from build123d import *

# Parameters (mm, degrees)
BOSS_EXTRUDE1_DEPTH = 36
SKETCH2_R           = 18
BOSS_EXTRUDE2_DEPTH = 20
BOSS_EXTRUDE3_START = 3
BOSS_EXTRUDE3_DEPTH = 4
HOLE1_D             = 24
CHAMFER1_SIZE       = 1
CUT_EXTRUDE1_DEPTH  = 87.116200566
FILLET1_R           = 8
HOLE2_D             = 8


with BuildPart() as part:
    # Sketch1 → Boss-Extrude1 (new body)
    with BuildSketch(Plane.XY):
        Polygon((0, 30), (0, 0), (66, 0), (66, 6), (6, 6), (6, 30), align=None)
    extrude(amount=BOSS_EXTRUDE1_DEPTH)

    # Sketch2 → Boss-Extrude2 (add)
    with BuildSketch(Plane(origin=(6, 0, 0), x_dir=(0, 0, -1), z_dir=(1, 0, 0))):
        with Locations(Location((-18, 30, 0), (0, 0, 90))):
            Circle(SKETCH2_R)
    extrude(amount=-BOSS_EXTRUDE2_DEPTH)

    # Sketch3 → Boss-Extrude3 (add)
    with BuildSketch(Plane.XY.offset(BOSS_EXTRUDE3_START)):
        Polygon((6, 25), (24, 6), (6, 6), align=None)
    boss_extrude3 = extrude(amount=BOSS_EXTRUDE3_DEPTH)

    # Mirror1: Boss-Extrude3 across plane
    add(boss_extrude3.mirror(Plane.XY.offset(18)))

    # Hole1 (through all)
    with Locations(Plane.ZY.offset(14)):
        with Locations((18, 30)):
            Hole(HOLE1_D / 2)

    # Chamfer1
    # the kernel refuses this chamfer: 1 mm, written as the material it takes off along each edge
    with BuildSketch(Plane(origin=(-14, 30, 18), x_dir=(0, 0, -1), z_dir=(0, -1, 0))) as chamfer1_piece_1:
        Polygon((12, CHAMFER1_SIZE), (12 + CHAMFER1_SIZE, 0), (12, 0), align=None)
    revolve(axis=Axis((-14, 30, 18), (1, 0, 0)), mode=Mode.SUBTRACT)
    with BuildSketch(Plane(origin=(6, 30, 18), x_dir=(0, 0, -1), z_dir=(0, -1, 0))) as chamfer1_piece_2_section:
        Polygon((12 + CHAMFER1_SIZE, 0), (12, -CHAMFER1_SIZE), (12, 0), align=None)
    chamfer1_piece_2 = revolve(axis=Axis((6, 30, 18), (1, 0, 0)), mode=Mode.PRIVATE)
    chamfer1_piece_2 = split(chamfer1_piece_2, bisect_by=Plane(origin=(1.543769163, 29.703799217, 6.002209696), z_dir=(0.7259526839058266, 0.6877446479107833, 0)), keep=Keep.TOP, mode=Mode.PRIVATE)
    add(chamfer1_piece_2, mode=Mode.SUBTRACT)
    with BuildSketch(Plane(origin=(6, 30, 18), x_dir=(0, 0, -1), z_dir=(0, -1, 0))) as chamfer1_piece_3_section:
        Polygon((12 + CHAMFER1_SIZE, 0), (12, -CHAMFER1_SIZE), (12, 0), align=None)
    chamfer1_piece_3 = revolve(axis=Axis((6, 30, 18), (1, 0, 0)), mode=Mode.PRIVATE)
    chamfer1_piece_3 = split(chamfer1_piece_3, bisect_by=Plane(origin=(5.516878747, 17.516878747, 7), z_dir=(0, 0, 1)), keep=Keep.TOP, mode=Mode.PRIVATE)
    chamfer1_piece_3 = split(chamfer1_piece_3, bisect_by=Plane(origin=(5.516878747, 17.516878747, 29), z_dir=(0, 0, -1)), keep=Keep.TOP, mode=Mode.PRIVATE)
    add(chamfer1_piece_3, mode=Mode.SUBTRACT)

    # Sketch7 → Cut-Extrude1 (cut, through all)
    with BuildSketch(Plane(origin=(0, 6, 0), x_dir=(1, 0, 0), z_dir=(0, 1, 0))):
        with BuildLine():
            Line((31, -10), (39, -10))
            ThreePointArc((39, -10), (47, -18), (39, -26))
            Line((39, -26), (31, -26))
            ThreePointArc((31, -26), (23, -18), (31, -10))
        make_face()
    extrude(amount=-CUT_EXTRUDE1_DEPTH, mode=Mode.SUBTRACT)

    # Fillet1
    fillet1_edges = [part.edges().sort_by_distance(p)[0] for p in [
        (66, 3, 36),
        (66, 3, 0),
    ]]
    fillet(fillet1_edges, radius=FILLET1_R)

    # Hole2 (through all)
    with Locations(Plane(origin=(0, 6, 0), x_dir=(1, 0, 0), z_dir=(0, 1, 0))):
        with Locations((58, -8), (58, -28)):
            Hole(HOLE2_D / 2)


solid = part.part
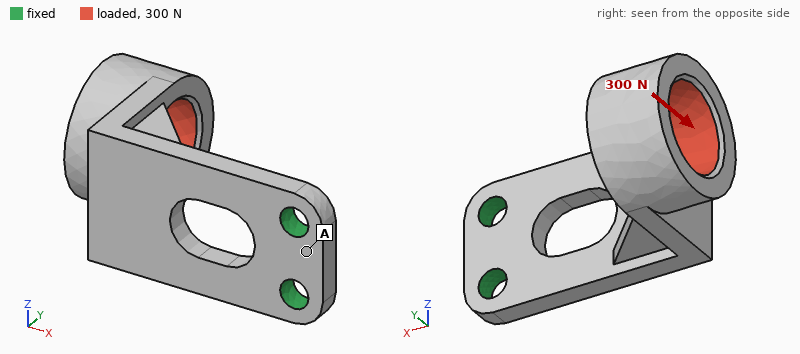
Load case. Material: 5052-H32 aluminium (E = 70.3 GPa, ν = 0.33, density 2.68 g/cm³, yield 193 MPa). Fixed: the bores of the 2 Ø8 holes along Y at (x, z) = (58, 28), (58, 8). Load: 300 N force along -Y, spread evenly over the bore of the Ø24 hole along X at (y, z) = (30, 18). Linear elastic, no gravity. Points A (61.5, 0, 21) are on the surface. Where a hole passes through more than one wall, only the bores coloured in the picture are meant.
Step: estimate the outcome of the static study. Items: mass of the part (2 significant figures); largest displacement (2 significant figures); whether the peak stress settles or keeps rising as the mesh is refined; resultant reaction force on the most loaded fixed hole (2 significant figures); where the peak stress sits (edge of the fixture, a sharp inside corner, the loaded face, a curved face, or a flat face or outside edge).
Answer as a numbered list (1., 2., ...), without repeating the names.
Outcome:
1. 70 g
2. 1.0 mm
3. keeps rising
4. 150 N
5. edge of the fixture
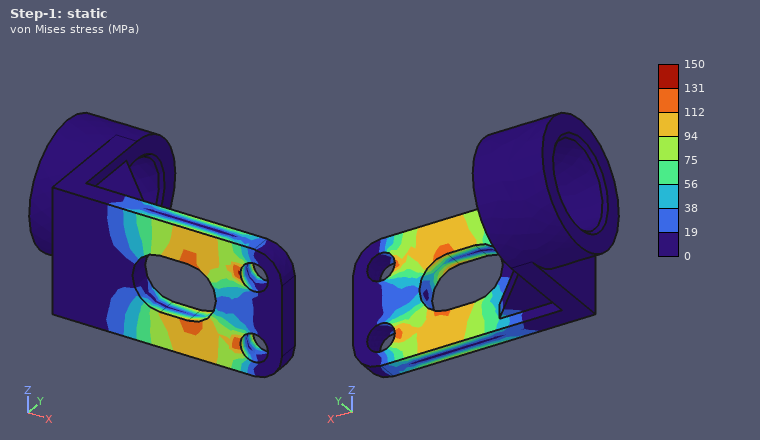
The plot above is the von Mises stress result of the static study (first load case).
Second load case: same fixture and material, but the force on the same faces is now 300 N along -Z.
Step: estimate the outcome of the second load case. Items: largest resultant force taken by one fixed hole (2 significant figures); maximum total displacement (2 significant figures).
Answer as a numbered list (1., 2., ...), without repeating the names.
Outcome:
1. 750 N
2. 0.26 mm
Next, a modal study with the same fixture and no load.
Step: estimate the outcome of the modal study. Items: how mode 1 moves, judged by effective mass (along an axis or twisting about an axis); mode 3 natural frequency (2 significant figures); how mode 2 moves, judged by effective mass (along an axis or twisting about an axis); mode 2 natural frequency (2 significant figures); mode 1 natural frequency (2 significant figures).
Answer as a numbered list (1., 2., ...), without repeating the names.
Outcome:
1. along Y
2. 2900 Hz
3. along Z
4. 1100 Hz
5. 460 Hz
